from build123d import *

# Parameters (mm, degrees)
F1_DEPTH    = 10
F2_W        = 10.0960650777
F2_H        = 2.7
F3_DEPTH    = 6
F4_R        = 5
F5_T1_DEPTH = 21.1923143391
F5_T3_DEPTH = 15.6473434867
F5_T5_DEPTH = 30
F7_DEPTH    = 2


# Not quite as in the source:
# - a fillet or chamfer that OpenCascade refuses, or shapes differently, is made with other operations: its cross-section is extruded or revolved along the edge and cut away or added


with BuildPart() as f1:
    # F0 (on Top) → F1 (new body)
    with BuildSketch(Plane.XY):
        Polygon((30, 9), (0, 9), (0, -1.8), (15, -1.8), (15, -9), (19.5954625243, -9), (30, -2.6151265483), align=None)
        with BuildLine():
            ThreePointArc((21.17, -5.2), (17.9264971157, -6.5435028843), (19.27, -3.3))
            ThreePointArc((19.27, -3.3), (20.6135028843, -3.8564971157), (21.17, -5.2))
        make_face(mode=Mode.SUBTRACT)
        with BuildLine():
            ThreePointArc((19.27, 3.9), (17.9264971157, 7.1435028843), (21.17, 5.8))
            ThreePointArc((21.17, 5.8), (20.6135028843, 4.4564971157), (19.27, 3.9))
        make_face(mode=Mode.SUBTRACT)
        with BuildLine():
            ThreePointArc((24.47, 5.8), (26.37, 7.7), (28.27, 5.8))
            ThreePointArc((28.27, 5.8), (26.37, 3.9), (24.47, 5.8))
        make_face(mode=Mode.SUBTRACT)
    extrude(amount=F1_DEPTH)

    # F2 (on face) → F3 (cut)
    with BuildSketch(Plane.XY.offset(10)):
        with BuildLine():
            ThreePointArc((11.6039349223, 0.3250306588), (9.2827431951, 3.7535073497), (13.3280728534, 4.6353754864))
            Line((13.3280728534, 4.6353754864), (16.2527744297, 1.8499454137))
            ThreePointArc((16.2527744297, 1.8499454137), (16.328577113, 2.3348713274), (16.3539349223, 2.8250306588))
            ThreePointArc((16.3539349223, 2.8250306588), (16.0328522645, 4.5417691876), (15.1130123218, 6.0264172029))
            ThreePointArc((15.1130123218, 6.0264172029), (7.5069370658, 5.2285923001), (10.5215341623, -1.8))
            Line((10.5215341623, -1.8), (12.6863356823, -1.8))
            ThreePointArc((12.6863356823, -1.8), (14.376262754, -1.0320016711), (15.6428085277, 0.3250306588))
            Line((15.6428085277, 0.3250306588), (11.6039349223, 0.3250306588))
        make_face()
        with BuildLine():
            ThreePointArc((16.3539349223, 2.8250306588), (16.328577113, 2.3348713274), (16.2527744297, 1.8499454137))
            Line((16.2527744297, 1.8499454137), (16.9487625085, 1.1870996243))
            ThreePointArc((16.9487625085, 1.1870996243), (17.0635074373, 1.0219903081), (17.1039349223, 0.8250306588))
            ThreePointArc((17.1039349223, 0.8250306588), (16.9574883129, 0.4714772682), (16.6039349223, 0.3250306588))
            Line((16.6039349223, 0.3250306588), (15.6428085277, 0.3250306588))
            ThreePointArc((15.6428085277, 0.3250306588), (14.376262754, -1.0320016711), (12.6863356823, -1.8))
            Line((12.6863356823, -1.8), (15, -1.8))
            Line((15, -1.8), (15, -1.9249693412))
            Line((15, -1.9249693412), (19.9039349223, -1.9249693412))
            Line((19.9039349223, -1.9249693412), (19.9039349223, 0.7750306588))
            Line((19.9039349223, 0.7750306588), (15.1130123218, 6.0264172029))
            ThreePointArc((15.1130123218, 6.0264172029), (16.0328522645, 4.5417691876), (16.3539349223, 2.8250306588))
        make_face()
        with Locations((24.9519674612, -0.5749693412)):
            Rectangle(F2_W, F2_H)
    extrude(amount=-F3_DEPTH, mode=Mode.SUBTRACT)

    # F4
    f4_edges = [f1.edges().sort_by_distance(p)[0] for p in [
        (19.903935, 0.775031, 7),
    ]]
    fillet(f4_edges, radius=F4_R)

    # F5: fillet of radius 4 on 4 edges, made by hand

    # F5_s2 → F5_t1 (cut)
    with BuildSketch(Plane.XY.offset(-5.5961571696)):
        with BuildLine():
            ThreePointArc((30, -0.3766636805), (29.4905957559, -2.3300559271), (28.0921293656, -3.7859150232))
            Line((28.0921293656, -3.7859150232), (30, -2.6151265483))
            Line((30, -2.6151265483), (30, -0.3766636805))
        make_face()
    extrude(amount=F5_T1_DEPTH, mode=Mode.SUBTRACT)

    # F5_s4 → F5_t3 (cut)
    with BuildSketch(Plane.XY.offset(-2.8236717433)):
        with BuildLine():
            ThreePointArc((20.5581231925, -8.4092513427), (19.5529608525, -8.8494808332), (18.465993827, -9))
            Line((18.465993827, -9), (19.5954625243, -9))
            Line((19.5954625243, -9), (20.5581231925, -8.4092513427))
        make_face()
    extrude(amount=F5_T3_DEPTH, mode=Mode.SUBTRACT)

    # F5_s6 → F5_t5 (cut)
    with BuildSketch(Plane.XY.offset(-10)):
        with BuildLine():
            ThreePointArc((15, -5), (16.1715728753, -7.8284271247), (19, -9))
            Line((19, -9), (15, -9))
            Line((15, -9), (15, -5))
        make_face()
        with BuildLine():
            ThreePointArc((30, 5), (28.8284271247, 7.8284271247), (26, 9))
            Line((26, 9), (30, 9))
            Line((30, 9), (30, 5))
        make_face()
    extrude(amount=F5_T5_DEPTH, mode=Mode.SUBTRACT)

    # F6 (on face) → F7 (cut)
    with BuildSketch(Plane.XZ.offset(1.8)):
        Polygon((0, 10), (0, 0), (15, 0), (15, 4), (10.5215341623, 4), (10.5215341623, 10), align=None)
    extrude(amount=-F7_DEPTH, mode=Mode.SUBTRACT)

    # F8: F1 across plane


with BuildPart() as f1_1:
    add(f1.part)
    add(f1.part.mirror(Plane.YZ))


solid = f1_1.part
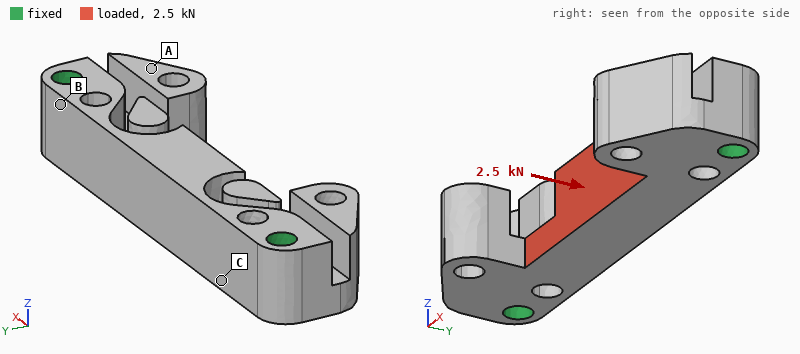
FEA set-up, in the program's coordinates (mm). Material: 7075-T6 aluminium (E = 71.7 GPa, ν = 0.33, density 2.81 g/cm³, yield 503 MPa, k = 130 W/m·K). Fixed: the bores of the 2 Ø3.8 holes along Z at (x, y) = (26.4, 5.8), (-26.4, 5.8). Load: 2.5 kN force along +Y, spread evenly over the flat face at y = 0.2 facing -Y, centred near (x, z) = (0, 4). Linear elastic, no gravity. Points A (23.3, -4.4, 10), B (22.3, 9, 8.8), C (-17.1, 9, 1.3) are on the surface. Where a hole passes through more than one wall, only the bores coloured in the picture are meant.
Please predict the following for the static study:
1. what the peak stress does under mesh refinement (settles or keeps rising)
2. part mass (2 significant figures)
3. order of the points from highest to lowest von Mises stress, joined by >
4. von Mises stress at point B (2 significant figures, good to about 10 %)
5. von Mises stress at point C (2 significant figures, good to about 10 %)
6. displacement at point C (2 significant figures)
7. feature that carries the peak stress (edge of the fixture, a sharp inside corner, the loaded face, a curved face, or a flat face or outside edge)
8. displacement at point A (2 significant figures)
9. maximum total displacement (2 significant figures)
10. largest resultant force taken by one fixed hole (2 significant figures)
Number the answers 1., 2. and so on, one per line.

1. keeps rising
2. 16 g
3. B > C > A
4. 73 MPa
5. 43 MPa
6. 0.032 mm
7. a sharp inside corner
8. 0.026 mm
9. 0.10 mm
10. 1.3 kN
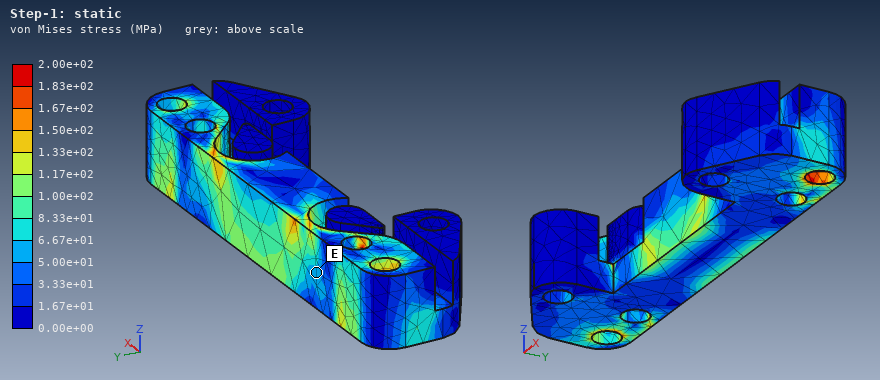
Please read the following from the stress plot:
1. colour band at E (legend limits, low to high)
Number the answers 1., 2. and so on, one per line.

1. 5.00e+01 to 6.67e+01 MPa
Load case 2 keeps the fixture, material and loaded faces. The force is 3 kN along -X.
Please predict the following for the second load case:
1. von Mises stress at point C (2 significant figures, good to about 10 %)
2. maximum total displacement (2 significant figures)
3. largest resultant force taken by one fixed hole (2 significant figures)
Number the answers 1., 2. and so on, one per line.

1. 34 MPa
2. 30 µm
3. 1.5 kN
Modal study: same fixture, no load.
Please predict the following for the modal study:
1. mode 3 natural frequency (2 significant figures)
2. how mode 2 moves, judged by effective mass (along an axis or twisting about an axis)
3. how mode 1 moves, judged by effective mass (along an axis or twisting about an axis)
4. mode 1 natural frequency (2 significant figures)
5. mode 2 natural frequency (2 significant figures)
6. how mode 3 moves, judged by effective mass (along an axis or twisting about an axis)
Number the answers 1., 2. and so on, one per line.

1. 15 kHz
2. along Z
3. along Y
4. 11 kHz
5. 11 kHz
6. twisting about X
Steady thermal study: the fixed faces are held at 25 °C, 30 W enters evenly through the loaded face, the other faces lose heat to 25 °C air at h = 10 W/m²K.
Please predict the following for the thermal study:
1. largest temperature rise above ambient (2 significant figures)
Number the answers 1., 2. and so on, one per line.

1. 44 K
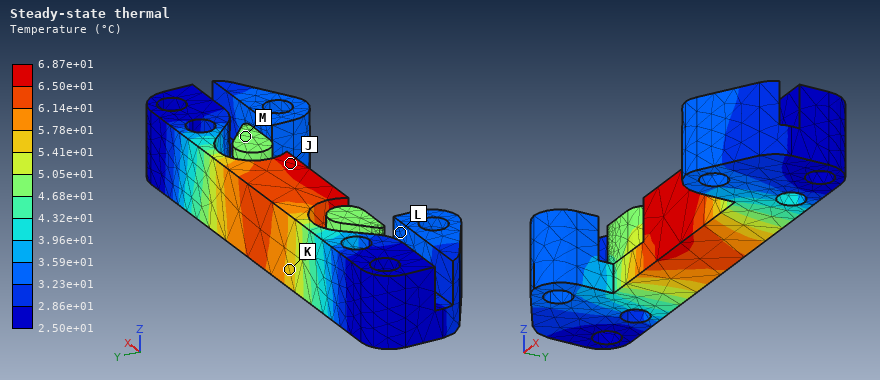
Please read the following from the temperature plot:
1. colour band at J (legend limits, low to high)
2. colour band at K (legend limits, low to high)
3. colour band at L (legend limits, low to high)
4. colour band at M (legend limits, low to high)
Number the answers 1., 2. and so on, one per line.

1. 6.50e+01 to 6.87e+01 °C
2. 5.41e+01 to 5.78e+01 °C
3. 3.23e+01 to 3.59e+01 °C
4. 4.68e+01 to 5.05e+01 °C
